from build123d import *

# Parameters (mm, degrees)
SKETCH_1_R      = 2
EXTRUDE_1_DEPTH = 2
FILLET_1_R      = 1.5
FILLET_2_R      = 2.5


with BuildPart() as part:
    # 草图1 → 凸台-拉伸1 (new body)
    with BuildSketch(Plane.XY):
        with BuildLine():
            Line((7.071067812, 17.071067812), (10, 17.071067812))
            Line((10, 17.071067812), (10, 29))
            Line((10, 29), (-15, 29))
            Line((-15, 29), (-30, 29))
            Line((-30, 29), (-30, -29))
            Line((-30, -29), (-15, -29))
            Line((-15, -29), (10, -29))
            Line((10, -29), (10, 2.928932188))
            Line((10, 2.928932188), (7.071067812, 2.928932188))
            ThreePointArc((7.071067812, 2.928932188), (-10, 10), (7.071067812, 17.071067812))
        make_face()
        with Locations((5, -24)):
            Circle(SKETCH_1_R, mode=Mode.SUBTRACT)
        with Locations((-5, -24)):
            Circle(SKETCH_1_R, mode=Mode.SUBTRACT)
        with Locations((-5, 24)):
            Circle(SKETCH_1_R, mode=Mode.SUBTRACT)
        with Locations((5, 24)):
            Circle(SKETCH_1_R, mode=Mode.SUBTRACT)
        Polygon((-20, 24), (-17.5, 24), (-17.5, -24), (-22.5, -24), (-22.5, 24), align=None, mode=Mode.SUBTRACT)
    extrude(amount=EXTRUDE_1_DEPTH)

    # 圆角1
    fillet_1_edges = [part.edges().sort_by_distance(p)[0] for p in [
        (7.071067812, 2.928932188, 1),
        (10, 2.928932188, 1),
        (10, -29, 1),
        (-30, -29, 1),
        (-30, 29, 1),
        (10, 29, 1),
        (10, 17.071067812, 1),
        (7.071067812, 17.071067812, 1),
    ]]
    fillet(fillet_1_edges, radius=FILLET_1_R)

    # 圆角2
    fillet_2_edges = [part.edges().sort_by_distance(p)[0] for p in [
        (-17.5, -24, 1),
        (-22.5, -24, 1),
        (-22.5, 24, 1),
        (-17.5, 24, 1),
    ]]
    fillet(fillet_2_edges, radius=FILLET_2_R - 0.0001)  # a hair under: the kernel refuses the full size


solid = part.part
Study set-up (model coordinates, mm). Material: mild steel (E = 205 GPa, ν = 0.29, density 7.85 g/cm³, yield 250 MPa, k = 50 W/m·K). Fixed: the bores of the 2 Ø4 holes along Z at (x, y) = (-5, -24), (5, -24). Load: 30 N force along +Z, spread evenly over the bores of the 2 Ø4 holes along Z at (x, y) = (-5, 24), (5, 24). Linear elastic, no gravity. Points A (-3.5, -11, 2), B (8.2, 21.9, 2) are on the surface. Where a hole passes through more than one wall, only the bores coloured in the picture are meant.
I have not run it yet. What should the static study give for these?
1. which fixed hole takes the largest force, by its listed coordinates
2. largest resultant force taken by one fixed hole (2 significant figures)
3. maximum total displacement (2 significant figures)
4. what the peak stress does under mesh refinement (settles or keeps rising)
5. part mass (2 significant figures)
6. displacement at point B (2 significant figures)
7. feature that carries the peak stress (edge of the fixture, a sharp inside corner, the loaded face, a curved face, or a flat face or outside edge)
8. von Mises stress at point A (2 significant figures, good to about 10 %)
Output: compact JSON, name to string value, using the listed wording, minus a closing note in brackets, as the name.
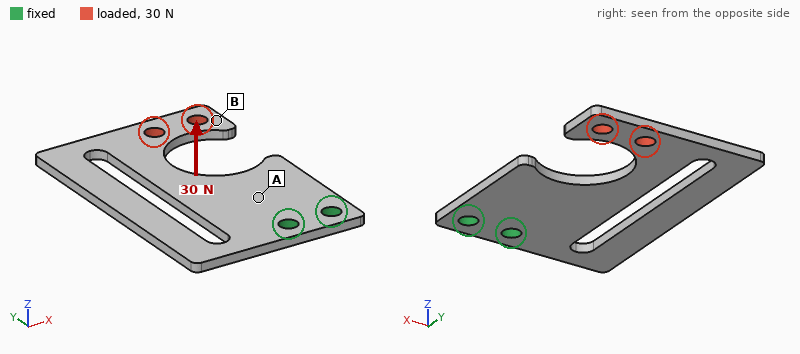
{"which fixed hole takes the largest force, by its listed coordinates": "(-5, -24)", "largest resultant force taken by one fixed hole": "25 N", "maximum total displacement": "0.52 mm", "what the peak stress does under mesh refinement": "keeps rising", "part mass": "27 g", "displacement at point B": "0.43 mm", "feature that carries the peak stress": "edge of the fixture", "von Mises stress at point A": "49 MPa"}
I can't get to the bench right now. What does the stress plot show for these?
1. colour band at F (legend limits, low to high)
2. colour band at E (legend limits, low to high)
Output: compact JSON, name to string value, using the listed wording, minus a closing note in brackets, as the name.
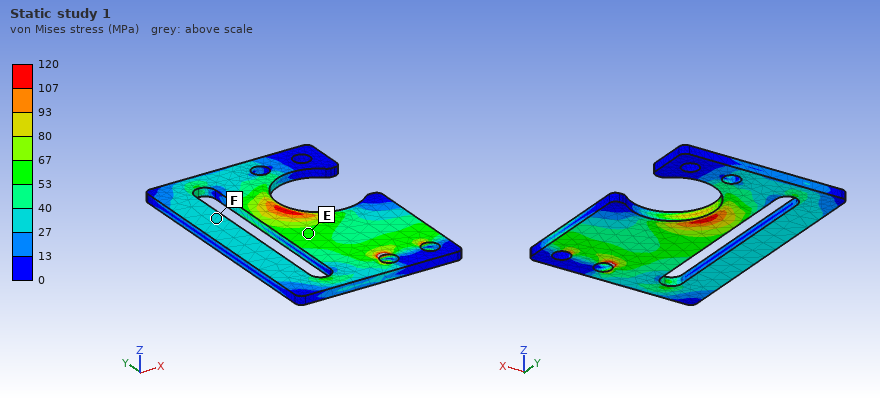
{"colour band at F": "27 to 40 MPa", "colour band at E": "53 to 67 MPa"}
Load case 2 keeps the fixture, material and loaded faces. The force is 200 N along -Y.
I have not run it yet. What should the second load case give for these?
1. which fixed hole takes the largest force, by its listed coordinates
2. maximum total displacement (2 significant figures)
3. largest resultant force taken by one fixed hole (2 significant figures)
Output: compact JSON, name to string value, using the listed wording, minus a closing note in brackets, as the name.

{"which fixed hole takes the largest force, by its listed coordinates": "(-5, -24)", "maximum total displacement": "54 µm", "largest resultant force taken by one fixed hole": "120 N"}
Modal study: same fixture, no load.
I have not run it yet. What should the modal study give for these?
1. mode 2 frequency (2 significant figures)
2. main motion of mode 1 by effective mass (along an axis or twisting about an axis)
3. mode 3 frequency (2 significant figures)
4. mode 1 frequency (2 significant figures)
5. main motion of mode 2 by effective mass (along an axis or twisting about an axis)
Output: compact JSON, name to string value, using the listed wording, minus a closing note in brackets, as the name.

{"mode 2 frequency": "1100 Hz", "main motion of mode 1 by effective mass": "along Z", "mode 3 frequency": "2400 Hz", "mode 1 frequency": "530 Hz", "main motion of mode 2 by effective mass": "twisting about Y"}
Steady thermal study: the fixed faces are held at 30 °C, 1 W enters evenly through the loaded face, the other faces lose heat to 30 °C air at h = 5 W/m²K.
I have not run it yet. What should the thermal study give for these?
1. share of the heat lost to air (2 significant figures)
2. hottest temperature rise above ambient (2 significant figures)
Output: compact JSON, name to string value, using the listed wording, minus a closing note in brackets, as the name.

{"share of the heat lost to air": "22 %", "hottest temperature rise above ambient": "37 K"}
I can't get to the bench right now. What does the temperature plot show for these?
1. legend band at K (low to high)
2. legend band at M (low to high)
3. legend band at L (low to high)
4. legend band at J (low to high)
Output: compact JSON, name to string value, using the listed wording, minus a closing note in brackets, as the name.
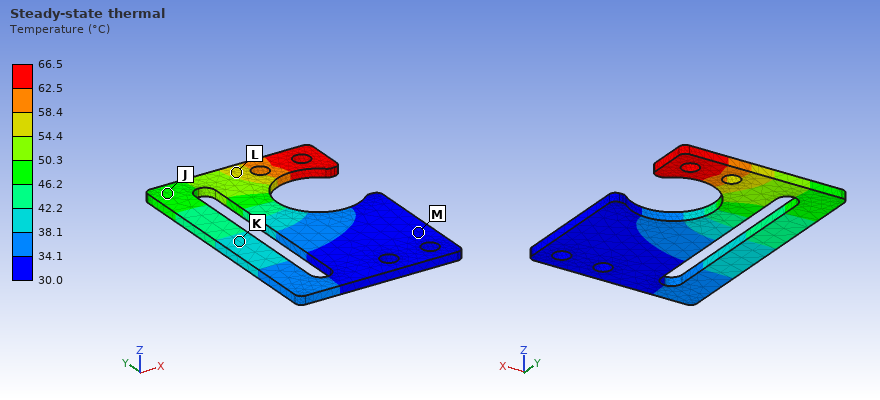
{"legend band at K": "38.1 to 42.2 °C", "legend band at M": "30.0 to 34.1 °C", "legend band at L": "54.4 to 58.4 °C", "legend band at J": "46.2 to 50.3 °C"}
